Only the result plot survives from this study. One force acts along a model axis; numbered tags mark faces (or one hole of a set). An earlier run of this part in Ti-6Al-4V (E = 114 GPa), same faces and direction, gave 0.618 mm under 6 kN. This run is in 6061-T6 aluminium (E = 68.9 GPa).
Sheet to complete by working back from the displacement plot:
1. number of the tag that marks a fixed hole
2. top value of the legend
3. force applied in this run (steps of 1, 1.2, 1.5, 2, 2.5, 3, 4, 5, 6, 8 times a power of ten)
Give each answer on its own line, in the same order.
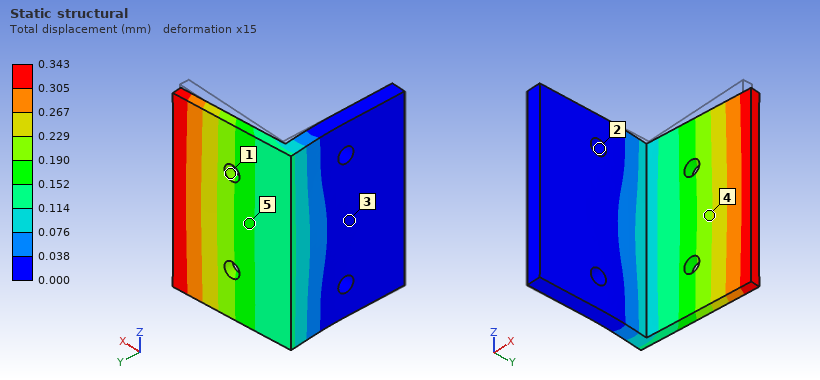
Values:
2
0.343 mm
2 kN
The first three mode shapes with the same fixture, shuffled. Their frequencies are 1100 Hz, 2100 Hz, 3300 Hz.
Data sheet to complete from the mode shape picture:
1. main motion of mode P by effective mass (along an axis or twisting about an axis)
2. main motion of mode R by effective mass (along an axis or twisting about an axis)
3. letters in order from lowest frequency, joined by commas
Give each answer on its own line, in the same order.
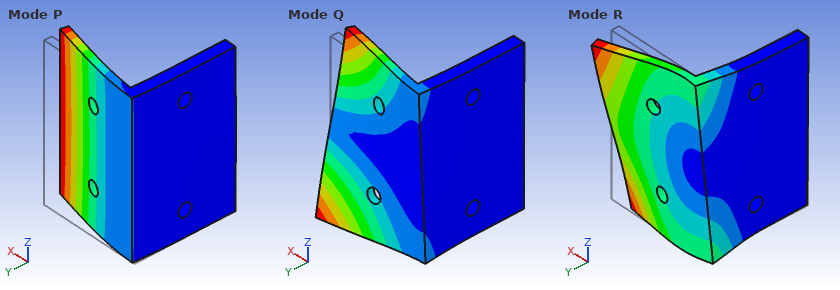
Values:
along Y
along Z
P, Q, R
